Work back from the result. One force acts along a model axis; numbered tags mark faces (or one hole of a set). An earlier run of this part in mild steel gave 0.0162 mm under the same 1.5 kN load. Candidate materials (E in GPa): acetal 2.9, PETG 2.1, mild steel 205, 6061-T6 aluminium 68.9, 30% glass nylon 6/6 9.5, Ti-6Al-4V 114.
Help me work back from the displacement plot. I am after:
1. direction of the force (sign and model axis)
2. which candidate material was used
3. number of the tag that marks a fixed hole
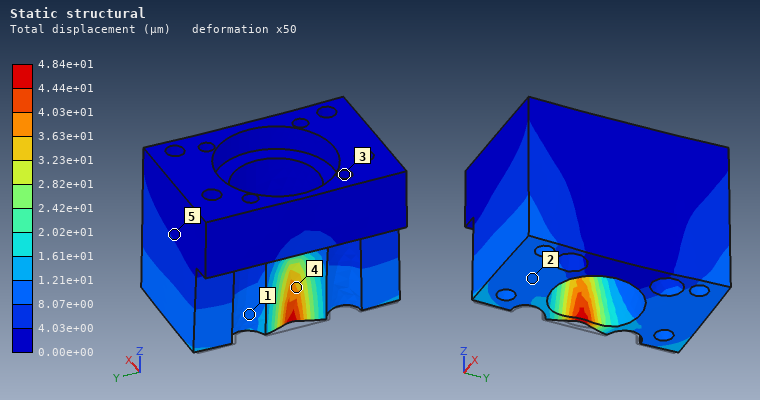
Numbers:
+X
6061-T6 aluminium
3
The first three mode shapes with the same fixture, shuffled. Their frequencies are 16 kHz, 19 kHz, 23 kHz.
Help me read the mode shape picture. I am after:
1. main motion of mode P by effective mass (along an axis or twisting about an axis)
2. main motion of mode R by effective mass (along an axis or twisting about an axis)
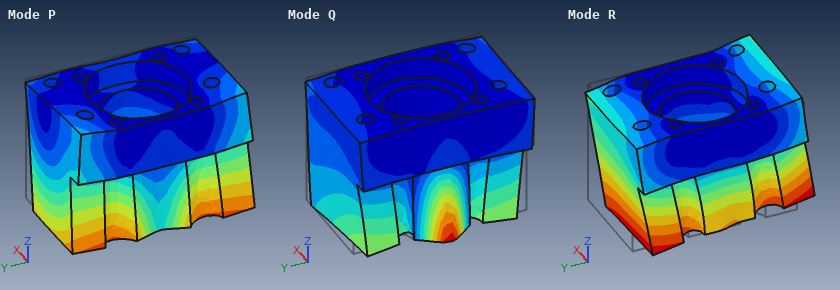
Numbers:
along X
along Y
